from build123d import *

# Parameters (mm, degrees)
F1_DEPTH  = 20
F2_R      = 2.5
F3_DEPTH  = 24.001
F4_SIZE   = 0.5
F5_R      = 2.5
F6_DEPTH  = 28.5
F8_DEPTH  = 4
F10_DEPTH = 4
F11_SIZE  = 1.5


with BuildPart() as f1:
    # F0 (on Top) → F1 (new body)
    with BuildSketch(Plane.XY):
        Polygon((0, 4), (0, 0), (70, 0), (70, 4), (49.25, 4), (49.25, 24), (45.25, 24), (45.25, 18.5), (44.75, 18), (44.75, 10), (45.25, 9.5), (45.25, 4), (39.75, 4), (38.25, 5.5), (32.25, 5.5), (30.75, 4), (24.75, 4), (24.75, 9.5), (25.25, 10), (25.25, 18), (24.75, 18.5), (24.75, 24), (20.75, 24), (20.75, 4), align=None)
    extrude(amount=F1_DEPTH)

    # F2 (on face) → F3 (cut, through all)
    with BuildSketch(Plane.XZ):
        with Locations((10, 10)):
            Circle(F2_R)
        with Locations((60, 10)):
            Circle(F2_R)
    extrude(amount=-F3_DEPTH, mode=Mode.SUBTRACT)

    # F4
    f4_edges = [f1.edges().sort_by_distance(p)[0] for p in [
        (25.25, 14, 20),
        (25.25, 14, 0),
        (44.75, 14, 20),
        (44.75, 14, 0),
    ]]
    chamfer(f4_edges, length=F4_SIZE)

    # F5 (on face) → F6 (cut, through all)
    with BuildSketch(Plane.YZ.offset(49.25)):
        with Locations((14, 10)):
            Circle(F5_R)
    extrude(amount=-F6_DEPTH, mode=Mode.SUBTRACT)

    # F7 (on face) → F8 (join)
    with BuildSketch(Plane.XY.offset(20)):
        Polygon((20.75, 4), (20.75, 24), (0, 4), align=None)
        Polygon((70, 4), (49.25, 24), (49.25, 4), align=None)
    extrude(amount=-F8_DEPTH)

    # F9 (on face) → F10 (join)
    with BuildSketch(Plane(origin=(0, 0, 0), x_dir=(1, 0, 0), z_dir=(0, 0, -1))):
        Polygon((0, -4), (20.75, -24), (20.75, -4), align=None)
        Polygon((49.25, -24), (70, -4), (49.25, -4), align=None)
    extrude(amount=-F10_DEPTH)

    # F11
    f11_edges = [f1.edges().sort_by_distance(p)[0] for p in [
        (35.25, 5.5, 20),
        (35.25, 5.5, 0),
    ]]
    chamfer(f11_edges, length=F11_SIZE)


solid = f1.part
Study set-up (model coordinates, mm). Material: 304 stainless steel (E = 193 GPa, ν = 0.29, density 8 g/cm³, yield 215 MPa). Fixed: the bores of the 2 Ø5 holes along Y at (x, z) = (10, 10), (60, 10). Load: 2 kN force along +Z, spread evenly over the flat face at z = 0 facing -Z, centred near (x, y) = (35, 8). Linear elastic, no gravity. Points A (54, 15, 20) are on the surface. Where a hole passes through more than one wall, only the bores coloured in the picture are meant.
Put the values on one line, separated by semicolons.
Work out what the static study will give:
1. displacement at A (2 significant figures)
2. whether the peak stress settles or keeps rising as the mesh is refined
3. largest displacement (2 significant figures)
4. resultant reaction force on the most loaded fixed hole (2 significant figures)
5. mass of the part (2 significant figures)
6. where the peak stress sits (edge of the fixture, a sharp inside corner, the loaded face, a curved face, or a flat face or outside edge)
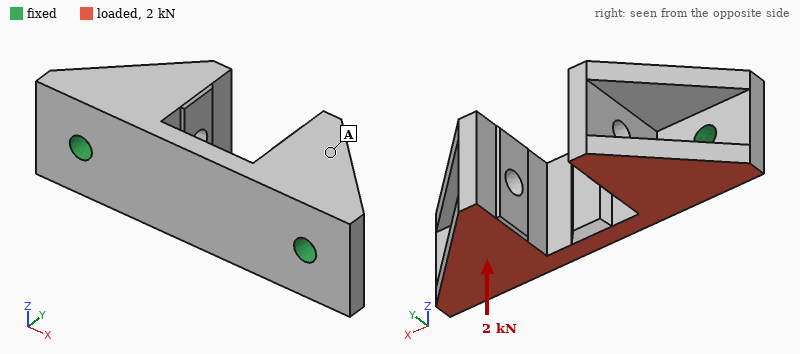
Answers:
15 µm; keeps rising; 25 µm; 1.0 kN; 97 g; edge of the fixture
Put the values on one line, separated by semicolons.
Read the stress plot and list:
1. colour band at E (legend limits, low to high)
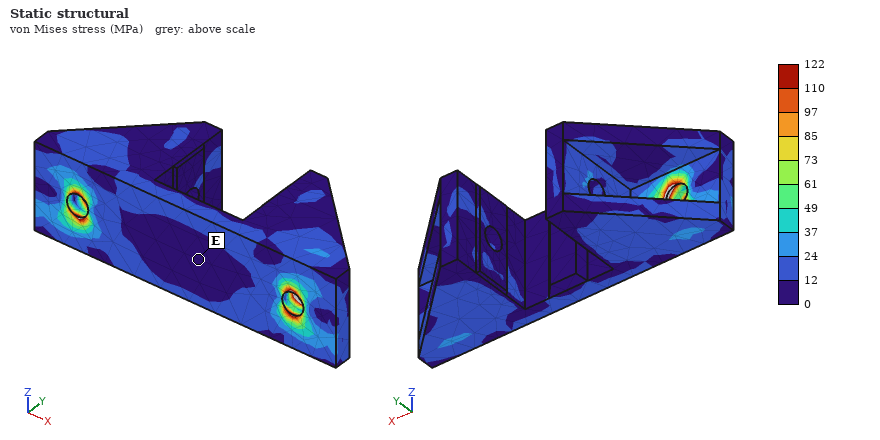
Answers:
0 to 12 MPa
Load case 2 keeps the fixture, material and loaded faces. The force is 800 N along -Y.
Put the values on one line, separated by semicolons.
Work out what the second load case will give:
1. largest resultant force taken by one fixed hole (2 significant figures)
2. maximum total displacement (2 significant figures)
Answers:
400 N; 14 µm
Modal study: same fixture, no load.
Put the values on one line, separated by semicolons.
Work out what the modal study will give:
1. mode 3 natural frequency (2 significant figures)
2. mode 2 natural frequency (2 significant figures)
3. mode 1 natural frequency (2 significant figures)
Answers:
7700 Hz; 5800 Hz; 5700 Hz
